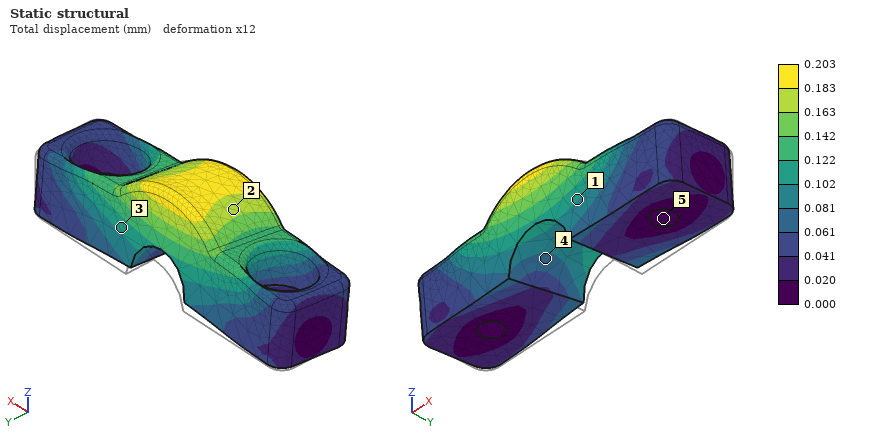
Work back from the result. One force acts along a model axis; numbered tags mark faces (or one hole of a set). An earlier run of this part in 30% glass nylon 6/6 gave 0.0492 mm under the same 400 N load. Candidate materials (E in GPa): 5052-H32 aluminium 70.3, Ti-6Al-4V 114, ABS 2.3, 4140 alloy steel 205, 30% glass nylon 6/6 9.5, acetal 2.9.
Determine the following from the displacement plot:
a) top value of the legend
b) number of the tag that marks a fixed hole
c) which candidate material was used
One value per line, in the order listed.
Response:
0.203 mm
5
ABS
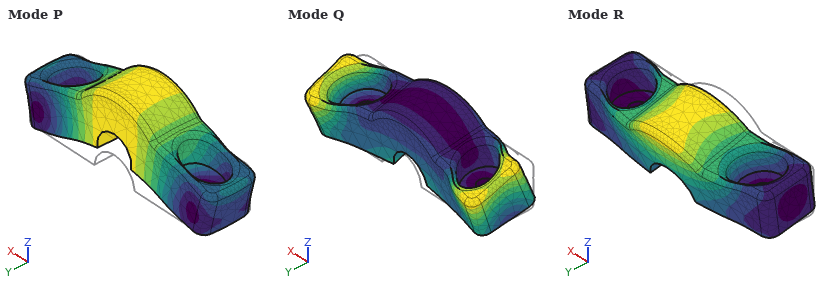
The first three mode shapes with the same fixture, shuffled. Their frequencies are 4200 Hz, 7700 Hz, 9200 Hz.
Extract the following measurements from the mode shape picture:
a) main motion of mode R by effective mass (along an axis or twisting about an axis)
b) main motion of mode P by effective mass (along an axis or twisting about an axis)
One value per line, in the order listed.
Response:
along Y
along Z
